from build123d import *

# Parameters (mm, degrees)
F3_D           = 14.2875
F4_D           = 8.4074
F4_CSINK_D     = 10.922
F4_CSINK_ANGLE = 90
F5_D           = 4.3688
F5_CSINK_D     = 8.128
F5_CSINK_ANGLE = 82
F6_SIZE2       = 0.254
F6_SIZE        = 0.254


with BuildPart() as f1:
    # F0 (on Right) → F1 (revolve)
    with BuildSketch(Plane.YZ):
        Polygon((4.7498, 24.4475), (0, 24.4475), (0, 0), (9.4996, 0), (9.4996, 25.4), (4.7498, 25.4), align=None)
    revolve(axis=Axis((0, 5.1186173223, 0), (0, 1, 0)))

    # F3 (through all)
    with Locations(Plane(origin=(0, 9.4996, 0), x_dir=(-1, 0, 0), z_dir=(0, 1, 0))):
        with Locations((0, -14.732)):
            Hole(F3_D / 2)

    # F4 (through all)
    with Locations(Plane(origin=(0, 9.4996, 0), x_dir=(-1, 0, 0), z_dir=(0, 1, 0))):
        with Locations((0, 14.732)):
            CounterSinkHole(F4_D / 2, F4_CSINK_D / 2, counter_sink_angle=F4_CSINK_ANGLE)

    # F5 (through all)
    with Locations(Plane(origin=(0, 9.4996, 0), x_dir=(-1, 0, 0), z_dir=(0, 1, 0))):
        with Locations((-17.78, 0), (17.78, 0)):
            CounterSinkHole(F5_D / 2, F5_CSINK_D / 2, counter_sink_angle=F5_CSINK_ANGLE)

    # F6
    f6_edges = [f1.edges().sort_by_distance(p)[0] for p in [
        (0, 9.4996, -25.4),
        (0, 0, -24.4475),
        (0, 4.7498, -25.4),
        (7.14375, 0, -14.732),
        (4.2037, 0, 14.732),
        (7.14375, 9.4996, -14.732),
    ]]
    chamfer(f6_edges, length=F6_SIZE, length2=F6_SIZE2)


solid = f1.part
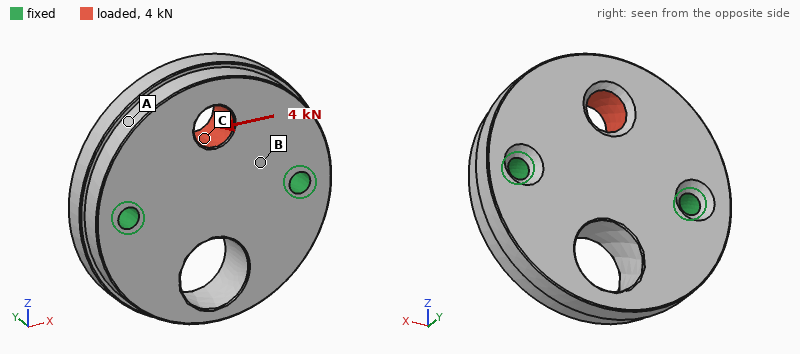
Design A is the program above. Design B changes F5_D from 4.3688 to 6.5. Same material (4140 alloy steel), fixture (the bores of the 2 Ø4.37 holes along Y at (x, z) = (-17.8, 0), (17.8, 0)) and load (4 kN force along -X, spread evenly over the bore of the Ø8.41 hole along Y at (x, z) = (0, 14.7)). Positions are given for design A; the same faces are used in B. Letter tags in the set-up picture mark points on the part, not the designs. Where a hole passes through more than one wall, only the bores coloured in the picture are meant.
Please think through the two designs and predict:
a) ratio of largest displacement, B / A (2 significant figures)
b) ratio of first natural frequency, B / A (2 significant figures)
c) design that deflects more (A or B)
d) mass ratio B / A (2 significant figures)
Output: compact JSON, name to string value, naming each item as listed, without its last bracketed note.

{"ratio of largest displacement, B / A": "0.88", "ratio of first natural frequency, B / A": "1.3", "design that deflects more": "A", "mass ratio B / A": "0.98"}
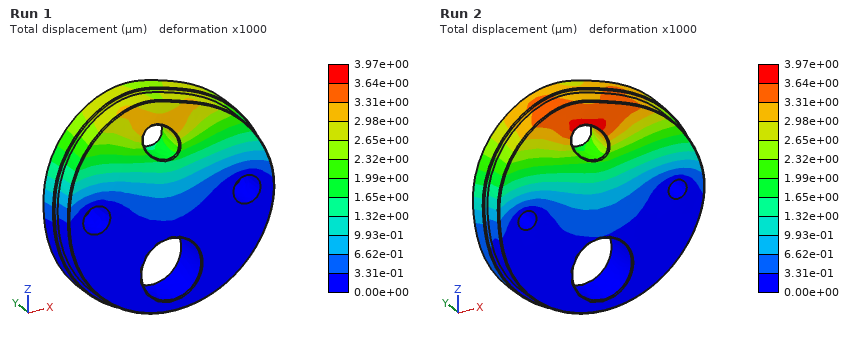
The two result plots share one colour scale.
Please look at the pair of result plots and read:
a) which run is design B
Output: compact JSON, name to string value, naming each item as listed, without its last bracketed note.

{"which run is design B": "Run 1"}
